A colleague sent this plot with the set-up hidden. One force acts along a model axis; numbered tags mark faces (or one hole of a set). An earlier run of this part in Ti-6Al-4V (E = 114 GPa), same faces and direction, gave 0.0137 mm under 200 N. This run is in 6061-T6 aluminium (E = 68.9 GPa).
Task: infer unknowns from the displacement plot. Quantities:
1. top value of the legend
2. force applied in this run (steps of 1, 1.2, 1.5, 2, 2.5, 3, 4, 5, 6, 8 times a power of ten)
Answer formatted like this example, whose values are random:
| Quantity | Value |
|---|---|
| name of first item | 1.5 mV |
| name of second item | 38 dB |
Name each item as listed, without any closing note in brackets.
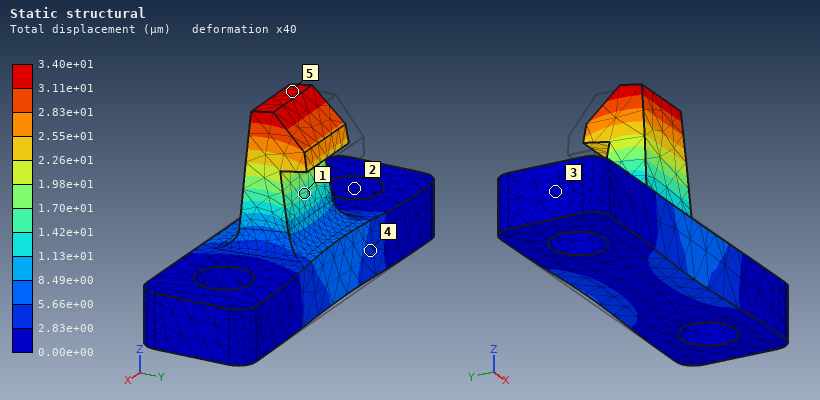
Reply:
| Quantity | Value |
|---|---|
| top value of the legend | 3.40e+01 µm |
| force applied in this run | 300 N |
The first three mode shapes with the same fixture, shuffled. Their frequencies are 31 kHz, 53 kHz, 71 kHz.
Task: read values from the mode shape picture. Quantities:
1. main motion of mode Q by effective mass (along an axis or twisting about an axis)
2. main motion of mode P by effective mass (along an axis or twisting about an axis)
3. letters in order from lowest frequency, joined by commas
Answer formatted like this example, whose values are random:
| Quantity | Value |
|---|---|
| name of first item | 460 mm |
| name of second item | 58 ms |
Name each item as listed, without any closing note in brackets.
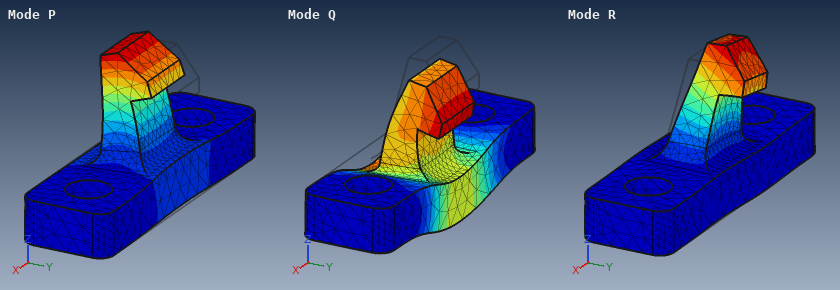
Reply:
| Quantity | Value |
|---|---|
| main motion of mode Q by effective mass | along Z |
| main motion of mode P by effective mass | along Y |
| letters in order from lowest frequency, joined by commas | P, R, Q |
